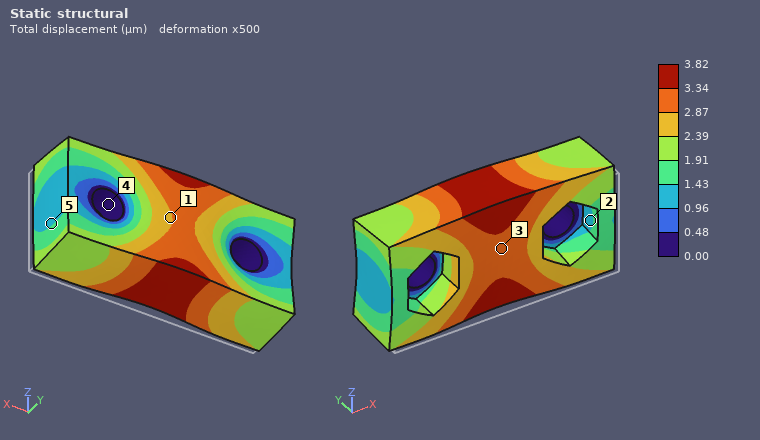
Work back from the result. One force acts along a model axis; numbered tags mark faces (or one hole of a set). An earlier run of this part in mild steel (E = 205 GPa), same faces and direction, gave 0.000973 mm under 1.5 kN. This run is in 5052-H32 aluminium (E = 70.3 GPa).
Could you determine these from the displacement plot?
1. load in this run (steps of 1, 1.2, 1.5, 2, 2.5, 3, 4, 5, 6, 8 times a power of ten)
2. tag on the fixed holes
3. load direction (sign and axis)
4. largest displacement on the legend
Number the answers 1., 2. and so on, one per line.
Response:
1. 2 kN
2. 4
3. +Y
4. 3.82 µm
